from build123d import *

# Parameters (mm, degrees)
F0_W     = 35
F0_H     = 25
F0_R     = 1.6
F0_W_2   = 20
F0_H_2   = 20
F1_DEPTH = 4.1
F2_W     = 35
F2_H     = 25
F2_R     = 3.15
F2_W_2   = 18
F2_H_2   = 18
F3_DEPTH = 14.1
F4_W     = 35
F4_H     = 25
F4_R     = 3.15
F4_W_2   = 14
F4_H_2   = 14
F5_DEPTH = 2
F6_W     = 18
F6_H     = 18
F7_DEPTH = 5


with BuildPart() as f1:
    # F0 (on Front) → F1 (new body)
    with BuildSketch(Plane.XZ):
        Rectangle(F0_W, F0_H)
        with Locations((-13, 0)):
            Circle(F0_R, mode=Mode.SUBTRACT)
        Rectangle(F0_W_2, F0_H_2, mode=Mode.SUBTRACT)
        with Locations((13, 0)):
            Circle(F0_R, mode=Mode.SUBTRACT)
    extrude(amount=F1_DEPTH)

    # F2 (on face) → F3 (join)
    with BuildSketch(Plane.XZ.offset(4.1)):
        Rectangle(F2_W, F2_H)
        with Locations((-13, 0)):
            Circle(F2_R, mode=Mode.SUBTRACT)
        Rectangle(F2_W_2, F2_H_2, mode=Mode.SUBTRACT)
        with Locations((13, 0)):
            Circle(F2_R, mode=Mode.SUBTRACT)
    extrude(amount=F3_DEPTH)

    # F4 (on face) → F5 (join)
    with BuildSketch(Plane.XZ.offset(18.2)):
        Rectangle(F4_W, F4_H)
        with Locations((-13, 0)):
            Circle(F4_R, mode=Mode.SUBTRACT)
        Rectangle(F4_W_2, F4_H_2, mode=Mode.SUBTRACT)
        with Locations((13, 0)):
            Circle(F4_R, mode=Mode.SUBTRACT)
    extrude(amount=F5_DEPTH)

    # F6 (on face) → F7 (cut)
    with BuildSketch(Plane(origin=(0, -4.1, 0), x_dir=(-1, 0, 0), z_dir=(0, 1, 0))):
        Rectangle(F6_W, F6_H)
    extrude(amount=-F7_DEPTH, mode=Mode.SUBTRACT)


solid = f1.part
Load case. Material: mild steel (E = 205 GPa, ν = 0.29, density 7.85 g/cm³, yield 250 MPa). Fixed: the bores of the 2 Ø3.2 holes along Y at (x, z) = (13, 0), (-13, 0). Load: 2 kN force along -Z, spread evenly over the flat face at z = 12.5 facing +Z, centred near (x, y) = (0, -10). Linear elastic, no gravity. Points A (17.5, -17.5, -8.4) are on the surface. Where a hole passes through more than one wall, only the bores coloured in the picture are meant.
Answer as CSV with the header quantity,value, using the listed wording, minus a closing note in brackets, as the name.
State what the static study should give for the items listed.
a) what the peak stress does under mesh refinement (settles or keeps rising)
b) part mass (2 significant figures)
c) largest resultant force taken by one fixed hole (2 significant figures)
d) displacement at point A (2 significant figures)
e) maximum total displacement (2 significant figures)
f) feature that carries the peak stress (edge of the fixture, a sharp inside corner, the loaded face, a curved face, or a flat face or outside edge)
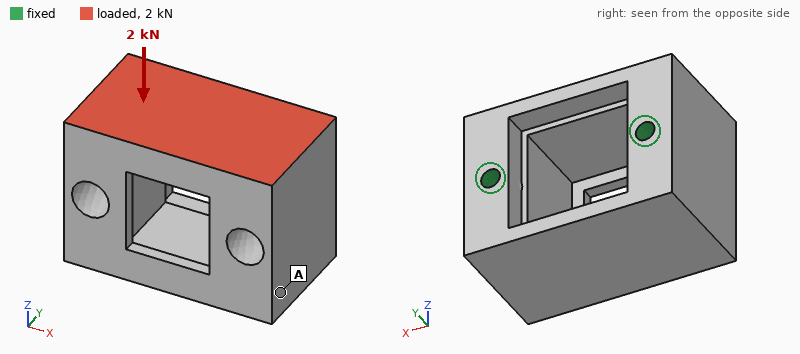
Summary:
quantity,value
what the peak stress does under mesh refinement,keeps rising
part mass,79 g
largest resultant force taken by one fixed hole,1.0 kN
displacement at point A,17 µm
maximum total displacement,23 µm
feature that carries the peak stress,edge of the fixture
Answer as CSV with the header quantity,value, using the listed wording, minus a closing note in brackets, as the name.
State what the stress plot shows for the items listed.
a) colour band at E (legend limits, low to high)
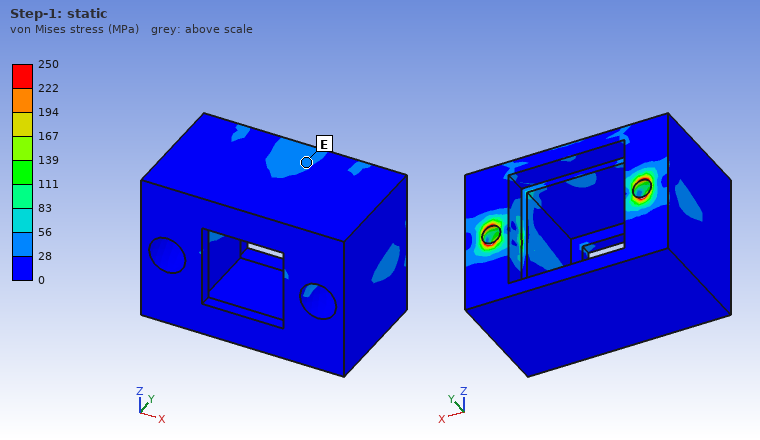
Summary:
quantity,value
colour band at E,28 to 56 MPa
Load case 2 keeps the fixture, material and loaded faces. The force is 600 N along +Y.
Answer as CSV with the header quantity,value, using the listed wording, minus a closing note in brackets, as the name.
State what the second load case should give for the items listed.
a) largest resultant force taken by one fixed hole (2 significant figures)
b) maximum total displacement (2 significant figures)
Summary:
quantity,value
largest resultant force taken by one fixed hole,300 N
maximum total displacement,10 µm
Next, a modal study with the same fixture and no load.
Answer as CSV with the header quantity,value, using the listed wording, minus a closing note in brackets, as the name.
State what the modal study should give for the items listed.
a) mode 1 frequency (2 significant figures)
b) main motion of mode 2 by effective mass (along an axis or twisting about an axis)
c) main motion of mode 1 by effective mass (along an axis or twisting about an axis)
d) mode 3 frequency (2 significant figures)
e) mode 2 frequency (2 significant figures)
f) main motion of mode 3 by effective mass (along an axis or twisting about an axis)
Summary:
quantity,value
mode 1 frequency,5600 Hz
main motion of mode 2 by effective mass,twisting about Y
main motion of mode 1 by effective mass,along Z
mode 3 frequency,13 kHz
mode 2 frequency,12 kHz
main motion of mode 3 by effective mass,along X
